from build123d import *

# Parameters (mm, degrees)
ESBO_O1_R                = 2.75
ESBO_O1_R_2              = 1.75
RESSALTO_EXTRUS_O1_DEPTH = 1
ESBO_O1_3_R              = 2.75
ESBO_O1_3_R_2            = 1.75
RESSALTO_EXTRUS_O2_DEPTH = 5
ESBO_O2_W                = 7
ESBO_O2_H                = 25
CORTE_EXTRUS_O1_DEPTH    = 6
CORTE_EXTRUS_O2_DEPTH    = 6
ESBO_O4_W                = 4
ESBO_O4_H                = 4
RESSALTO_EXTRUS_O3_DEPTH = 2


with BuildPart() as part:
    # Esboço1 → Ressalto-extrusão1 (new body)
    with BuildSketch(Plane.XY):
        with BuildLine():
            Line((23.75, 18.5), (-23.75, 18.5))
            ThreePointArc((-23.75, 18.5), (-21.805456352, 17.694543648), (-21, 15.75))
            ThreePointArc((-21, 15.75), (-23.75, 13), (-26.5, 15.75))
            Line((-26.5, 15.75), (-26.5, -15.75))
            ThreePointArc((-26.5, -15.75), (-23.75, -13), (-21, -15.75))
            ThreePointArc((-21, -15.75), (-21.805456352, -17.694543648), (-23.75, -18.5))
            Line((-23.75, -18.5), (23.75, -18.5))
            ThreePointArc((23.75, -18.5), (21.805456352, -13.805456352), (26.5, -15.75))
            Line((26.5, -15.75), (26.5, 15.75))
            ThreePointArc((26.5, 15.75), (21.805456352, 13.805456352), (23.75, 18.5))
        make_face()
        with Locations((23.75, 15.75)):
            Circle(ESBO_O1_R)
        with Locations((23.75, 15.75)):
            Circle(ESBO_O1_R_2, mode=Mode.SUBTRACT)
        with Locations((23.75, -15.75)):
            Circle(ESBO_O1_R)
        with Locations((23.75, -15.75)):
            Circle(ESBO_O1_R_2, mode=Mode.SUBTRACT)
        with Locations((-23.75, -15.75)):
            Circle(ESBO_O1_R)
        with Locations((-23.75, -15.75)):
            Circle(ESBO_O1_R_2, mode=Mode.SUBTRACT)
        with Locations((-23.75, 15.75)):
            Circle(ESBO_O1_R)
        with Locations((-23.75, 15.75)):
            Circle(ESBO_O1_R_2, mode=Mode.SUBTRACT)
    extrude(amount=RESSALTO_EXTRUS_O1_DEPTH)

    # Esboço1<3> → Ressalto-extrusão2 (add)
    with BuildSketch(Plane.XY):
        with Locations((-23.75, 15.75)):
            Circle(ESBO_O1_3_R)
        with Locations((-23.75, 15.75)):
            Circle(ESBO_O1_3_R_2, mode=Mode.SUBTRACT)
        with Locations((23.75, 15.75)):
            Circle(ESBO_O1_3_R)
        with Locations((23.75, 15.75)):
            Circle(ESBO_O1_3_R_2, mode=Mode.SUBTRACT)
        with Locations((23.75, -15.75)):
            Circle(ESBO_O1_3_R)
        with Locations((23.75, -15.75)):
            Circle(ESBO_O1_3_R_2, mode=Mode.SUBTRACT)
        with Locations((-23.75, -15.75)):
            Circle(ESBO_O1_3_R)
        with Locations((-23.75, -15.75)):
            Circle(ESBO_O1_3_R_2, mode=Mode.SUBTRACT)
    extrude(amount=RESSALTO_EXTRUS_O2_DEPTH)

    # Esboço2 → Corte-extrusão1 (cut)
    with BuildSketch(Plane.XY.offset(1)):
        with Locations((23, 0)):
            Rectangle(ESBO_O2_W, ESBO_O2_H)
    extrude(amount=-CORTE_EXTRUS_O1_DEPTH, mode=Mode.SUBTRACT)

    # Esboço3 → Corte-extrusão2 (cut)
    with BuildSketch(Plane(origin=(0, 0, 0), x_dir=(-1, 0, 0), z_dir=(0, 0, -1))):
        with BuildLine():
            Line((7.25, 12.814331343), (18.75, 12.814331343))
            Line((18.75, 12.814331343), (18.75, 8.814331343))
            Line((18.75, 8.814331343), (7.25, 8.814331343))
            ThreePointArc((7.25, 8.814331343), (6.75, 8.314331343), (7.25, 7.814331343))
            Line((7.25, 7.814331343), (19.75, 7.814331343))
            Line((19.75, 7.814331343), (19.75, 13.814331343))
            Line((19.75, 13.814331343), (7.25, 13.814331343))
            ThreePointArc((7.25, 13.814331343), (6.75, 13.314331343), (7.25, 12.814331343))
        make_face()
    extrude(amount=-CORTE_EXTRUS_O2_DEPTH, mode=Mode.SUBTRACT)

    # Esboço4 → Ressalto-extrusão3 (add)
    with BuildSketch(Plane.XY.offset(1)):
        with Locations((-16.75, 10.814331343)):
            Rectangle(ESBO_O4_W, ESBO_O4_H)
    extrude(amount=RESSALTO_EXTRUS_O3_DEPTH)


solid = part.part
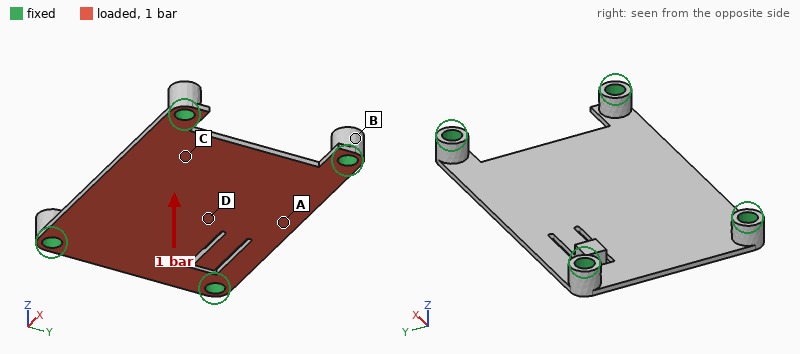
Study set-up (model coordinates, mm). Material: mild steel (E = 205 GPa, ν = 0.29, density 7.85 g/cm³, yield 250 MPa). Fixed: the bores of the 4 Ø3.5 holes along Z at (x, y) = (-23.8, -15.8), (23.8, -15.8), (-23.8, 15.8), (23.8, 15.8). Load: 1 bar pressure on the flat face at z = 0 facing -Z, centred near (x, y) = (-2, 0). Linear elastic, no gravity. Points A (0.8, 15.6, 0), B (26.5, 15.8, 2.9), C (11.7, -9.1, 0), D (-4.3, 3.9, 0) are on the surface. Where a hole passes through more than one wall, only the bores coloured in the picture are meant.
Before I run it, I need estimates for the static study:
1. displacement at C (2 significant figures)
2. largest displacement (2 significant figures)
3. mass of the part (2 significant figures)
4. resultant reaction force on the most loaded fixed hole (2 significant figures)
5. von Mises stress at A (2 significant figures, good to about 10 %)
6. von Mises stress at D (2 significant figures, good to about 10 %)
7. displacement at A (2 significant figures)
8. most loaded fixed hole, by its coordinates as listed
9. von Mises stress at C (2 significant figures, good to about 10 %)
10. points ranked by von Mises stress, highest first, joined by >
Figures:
0.061 mm
0.10 mm
15 g
53 N
64 MPa
52 MPa
0.094 mm
(-23.8, -15.8)
30 MPa
A > D > C > B
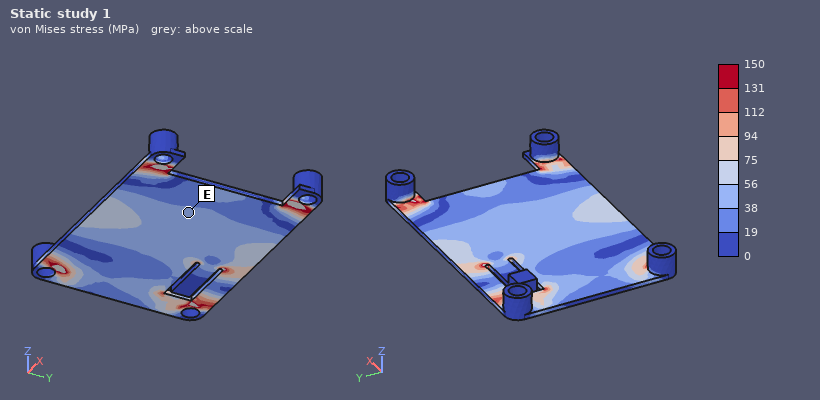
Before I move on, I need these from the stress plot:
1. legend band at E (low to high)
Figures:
38 to 56 MPa
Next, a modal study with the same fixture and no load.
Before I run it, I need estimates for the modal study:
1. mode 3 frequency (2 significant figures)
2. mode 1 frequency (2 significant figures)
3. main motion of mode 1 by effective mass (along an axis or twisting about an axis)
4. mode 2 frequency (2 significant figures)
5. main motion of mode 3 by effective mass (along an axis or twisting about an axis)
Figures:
3400 Hz
1900 Hz
along Z
2500 Hz
twisting about X
